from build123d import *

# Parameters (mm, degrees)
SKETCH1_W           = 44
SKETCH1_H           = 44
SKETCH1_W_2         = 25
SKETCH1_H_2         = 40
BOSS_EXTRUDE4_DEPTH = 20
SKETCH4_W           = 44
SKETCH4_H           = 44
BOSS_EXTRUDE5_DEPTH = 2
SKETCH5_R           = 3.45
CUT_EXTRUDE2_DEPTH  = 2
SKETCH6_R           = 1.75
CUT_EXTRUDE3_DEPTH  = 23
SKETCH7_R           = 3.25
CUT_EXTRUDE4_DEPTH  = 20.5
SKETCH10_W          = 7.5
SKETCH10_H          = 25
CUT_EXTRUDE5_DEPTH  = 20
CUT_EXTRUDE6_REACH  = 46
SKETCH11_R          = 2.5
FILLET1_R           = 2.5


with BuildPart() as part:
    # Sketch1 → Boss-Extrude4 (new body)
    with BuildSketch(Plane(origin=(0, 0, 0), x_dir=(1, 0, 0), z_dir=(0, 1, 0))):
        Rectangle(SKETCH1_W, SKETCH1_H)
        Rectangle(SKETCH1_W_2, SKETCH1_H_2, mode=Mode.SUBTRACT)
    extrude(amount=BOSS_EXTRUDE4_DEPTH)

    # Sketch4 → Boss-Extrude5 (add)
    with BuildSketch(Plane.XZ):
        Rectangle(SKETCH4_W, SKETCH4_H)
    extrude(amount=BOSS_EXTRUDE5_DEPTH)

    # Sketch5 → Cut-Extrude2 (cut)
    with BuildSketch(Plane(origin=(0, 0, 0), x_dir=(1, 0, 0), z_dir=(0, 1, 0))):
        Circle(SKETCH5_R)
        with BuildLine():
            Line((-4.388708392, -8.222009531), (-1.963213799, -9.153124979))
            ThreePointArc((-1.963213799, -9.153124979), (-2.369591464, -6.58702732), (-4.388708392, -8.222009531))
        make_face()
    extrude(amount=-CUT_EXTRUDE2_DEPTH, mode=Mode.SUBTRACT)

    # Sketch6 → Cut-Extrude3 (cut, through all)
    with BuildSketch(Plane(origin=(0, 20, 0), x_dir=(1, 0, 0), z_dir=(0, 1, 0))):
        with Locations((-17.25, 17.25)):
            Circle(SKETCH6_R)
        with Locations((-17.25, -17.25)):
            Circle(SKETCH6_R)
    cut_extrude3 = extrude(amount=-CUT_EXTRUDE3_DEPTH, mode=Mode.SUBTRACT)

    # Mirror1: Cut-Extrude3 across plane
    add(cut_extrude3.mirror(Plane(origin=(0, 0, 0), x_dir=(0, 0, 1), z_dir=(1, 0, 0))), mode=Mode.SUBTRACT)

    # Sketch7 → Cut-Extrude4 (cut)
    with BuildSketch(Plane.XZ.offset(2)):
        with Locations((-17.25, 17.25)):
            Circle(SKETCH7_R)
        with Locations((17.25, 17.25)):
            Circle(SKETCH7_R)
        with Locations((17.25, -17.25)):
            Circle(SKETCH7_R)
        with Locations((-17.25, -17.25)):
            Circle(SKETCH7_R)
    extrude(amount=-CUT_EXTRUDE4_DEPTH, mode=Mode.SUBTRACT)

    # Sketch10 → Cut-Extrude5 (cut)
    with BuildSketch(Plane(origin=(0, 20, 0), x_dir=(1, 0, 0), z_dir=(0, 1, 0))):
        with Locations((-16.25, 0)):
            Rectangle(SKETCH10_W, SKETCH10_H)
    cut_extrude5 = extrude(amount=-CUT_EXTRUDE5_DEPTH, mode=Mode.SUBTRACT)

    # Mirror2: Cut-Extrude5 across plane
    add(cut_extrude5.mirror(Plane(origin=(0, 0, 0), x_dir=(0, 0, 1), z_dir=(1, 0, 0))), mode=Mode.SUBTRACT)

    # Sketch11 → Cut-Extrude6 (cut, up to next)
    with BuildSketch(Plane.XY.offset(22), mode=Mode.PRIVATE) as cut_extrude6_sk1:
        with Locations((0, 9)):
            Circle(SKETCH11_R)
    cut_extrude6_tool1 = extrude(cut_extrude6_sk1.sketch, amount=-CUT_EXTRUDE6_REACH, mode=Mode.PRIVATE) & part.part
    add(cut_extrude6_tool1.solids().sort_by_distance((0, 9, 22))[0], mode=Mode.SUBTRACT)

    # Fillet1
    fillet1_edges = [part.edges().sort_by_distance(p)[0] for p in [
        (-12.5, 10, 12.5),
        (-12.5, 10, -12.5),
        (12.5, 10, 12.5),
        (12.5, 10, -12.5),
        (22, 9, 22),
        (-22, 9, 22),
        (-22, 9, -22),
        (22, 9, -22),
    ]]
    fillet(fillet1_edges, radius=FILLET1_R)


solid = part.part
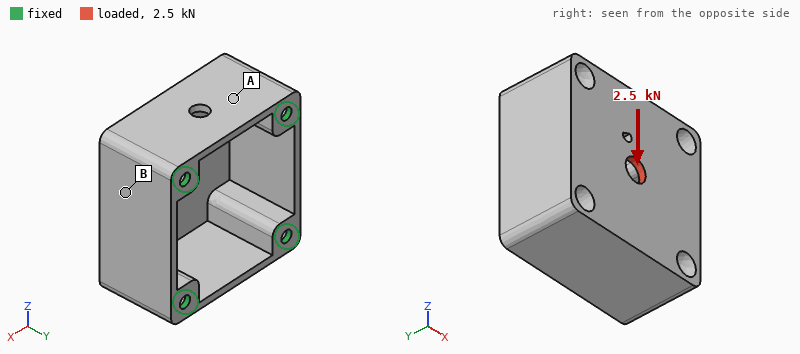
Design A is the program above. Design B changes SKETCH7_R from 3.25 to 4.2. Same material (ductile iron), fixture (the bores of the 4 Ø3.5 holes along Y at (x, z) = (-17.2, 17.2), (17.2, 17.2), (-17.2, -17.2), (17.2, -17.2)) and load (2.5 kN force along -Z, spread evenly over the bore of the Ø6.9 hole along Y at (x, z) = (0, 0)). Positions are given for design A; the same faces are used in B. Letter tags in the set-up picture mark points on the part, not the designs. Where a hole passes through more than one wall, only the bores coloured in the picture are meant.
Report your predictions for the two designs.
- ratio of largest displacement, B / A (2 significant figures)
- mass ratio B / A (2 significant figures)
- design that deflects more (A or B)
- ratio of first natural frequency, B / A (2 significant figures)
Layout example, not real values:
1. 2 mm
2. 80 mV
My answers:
1. 1.3
2. 0.85
3. B
4. 0.91
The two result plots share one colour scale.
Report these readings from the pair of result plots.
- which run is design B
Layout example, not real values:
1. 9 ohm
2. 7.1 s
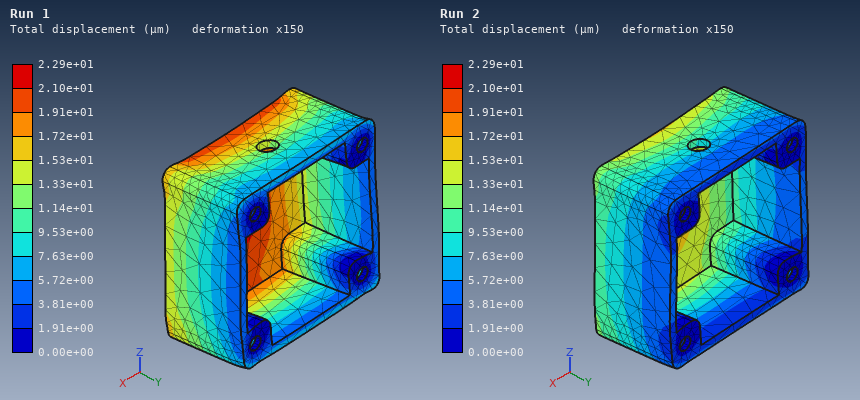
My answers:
1. Run 1
